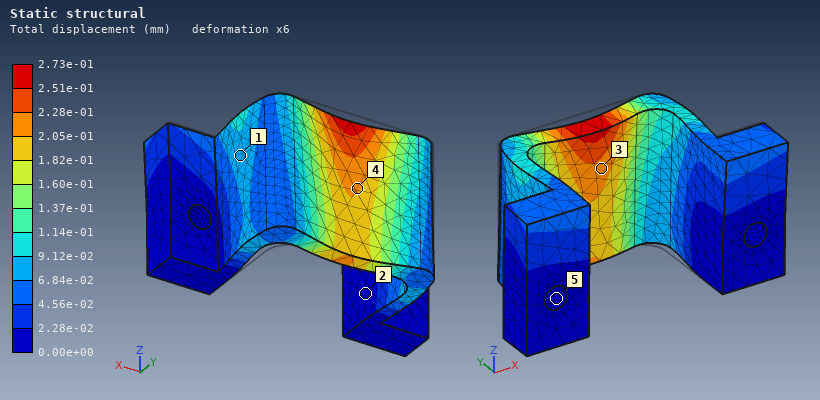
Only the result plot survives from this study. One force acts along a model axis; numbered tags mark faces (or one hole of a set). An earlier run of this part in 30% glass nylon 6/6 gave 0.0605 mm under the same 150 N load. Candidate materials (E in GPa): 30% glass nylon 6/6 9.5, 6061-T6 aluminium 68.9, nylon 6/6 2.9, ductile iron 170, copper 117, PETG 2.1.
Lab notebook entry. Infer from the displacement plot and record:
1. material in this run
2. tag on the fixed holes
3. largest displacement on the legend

PETG
5
2.73e-01 mm
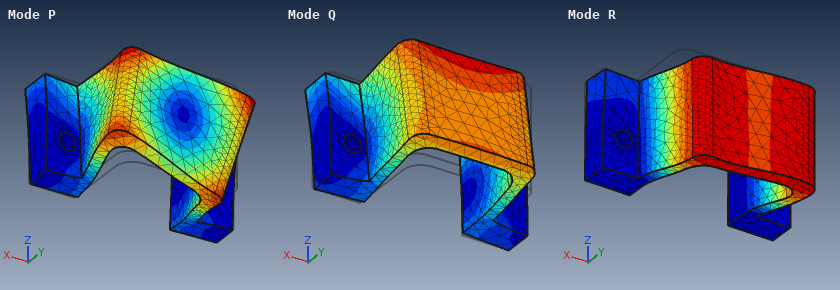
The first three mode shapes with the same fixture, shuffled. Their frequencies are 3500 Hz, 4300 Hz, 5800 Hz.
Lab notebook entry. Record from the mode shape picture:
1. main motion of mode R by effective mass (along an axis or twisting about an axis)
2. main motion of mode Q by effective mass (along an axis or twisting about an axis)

along X
along Z
